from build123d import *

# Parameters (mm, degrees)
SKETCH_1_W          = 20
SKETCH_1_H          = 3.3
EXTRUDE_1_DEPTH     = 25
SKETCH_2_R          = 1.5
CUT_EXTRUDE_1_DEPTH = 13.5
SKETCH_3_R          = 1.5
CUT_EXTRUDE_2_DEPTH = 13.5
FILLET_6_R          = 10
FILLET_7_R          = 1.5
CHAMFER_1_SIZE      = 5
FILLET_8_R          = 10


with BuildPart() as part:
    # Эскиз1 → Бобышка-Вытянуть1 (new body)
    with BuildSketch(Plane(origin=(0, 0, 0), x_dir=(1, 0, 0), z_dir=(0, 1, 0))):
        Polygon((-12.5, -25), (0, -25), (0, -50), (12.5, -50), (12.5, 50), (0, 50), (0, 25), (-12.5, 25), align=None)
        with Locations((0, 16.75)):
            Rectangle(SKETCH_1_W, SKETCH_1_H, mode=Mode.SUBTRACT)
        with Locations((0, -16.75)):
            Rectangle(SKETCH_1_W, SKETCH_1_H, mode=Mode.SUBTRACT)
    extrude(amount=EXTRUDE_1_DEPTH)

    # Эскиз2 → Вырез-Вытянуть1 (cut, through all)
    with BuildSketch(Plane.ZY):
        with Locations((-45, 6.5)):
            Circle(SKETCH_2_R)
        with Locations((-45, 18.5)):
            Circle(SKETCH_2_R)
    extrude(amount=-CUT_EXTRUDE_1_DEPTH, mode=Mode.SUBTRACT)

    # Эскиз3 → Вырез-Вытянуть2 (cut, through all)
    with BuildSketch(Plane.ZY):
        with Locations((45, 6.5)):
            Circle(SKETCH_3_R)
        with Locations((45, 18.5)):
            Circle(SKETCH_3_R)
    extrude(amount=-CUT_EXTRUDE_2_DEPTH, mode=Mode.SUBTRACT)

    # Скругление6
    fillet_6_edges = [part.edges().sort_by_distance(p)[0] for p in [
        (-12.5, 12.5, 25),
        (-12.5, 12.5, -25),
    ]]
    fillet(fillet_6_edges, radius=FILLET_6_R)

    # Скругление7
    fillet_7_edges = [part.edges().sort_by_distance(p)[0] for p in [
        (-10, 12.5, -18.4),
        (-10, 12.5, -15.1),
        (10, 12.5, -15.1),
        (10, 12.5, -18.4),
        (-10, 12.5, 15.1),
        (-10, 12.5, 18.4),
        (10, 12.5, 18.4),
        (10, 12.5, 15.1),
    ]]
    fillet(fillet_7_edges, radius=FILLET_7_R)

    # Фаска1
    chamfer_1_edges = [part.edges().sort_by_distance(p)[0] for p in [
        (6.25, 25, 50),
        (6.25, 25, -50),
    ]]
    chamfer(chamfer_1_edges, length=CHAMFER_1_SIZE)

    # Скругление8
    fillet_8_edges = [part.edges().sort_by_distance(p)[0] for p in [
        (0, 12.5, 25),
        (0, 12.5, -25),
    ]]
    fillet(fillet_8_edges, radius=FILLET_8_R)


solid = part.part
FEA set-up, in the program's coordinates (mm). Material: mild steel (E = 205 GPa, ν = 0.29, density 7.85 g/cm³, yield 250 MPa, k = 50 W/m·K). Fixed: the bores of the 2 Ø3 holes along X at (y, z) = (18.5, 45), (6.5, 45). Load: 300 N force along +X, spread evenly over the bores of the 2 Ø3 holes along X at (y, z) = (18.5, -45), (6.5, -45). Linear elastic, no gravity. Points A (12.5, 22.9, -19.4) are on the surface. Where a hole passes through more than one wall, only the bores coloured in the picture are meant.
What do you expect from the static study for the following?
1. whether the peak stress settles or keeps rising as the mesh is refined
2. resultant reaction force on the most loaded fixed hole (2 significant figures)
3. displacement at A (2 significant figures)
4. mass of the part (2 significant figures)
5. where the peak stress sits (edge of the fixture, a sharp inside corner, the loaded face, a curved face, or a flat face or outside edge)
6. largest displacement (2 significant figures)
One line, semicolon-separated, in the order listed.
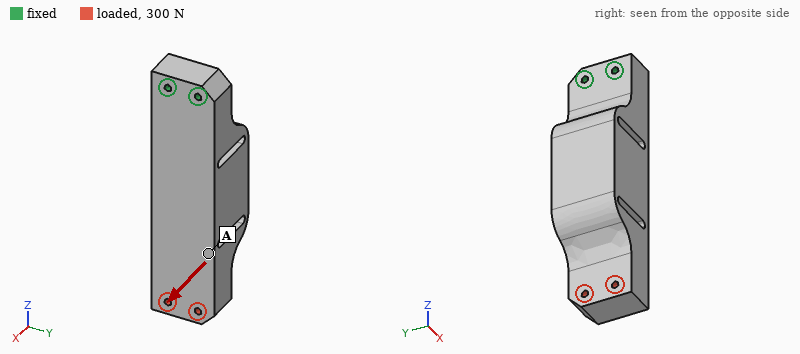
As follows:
keeps rising; 160 N; 44 µm; 330 g; edge of the fixture; 72 µm
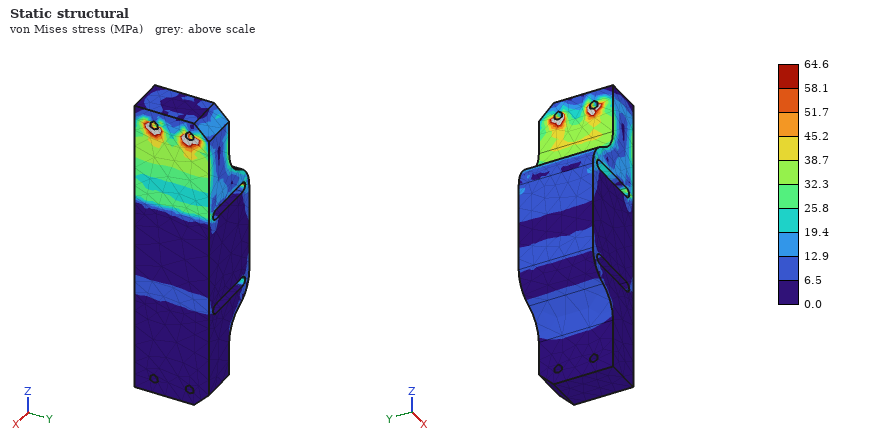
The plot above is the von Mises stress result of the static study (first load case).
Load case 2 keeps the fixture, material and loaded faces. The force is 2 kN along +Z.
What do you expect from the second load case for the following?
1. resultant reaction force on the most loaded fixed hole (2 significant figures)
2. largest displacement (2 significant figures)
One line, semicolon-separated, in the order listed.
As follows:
1.0 kN; 5.3 µm
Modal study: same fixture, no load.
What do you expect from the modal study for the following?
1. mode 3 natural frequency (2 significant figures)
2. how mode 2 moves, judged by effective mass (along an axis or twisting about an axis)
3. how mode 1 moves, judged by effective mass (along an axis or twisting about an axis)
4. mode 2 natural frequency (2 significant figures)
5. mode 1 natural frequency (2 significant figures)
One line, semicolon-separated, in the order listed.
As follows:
5300 Hz; along Y; along X; 1600 Hz; 1100 Hz
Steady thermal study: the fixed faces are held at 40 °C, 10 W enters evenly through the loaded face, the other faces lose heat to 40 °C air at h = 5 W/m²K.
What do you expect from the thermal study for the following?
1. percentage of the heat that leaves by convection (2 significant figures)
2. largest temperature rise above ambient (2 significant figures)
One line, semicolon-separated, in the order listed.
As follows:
16 %; 59 K
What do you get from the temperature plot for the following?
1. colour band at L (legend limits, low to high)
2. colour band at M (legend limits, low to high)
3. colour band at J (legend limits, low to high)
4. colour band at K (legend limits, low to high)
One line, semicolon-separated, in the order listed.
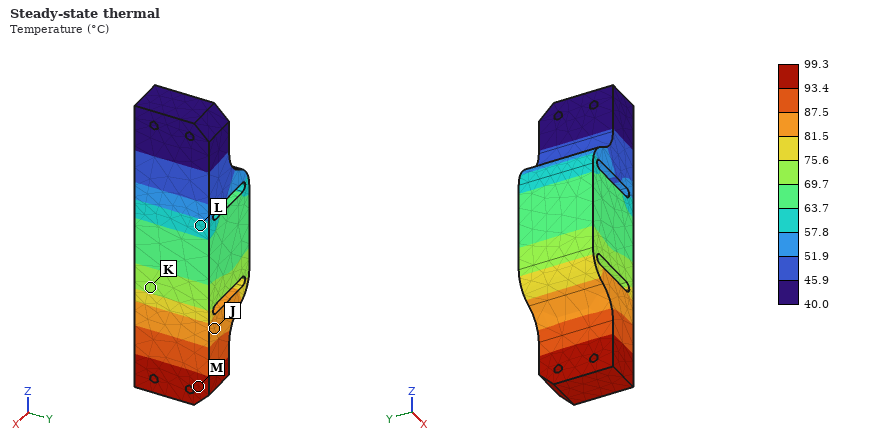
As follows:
57.8 to 63.7 °C; 93.4 to 99.3 °C; 81.5 to 87.5 °C; 69.7 to 75.6 °C
